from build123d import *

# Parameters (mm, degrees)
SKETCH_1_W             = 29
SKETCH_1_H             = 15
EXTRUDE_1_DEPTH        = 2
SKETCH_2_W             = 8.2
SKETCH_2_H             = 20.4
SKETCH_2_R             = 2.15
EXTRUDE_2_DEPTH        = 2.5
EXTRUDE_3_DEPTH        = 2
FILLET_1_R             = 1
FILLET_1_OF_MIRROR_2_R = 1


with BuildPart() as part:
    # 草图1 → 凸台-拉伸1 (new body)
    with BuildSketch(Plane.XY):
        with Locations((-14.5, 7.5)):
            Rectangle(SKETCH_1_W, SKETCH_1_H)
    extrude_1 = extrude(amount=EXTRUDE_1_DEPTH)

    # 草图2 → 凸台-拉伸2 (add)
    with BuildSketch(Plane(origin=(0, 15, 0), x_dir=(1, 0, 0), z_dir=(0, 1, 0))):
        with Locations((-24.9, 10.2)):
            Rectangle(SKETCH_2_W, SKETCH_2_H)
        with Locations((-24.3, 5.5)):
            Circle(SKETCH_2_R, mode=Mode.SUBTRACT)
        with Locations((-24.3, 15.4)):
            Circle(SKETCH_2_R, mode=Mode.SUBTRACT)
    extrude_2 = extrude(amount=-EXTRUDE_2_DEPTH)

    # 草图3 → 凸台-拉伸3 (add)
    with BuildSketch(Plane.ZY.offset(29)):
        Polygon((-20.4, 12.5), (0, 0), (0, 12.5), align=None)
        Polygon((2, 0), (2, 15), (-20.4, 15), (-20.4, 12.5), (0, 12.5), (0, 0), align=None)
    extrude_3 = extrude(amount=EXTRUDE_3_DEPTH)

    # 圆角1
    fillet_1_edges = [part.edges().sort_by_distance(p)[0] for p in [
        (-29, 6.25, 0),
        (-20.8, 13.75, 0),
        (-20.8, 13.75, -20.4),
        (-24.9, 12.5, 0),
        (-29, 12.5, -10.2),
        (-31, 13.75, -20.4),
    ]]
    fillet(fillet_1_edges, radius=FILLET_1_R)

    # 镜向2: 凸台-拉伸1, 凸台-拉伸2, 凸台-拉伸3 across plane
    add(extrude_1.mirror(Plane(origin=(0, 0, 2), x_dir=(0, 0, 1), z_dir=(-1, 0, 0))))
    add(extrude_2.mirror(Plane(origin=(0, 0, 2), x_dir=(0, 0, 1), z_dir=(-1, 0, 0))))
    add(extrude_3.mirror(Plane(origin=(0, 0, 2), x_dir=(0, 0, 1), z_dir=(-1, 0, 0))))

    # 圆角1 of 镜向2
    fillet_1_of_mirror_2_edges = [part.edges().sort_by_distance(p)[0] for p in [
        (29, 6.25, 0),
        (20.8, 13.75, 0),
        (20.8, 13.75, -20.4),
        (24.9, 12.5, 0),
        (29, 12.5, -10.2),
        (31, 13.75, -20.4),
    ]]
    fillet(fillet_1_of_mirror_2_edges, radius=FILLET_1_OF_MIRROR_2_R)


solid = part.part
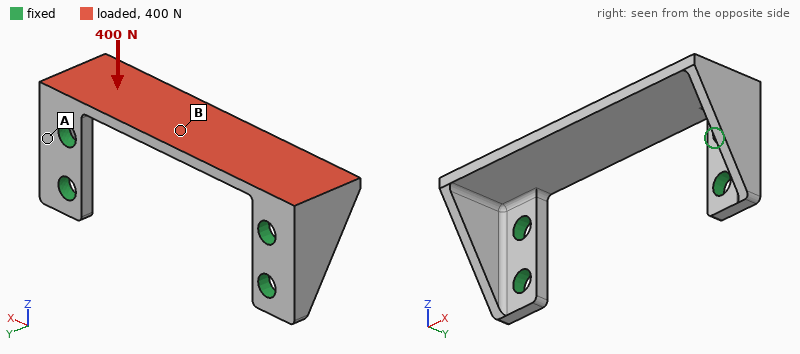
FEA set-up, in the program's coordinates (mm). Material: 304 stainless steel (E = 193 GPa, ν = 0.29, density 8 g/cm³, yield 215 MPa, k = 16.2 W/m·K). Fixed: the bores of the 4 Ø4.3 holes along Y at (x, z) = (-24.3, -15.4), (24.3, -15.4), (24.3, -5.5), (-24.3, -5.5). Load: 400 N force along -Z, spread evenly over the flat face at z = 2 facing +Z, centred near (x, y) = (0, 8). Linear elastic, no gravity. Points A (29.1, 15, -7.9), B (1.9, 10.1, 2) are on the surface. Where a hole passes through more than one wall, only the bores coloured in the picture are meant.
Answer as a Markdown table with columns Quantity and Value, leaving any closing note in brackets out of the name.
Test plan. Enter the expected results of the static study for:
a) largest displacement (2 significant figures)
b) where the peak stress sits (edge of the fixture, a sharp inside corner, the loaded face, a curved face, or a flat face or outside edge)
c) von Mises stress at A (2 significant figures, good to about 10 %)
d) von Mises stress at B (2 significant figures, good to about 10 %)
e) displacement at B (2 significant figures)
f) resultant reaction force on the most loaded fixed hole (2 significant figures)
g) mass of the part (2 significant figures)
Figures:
| Quantity | Value |
|---|---|
| largest displacement | 83 µm |
| where the peak stress sits | a curved face |
| von Mises stress at A | 18 MPa |
| von Mises stress at B | 68 MPa |
| displacement at B | 54 µm |
| resultant reaction force on the most loaded fixed hole | 220 N |
| mass of the part | 26 g |
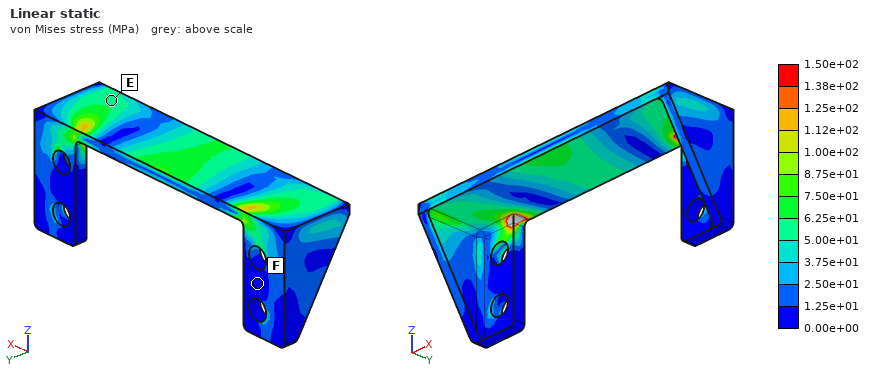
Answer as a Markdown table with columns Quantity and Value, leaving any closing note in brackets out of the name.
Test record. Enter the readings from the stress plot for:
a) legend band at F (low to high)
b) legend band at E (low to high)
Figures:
| Quantity | Value |
|---|---|
| legend band at F | 0.00e+00 to 1.25e+01 MPa |
| legend band at E | 5.00e+01 to 6.25e+01 MPa |
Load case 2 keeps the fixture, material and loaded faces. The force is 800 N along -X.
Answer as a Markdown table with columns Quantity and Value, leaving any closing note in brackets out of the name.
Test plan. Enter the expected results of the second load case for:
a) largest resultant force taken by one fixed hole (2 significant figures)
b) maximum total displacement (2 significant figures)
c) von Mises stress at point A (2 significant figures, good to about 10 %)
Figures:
| Quantity | Value |
|---|---|
| largest resultant force taken by one fixed hole | 490 N |
| maximum total displacement | 6.3 µm |
| von Mises stress at point A | 24 MPa |
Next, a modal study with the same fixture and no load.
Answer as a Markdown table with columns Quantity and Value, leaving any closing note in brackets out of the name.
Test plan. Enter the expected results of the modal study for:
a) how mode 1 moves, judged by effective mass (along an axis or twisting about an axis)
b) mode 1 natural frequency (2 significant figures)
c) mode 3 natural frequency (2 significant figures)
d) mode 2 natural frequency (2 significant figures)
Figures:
| Quantity | Value |
|---|---|
| how mode 1 moves, judged by effective mass | along Z |
| mode 1 natural frequency | 3700 Hz |
| mode 3 natural frequency | 8900 Hz |
| mode 2 natural frequency | 8500 Hz |
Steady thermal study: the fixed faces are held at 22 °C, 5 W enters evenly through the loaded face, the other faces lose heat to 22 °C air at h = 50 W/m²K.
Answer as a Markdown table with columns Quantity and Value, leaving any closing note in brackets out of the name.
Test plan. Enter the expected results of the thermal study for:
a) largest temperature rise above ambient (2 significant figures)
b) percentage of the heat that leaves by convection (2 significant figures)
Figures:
| Quantity | Value |
|---|---|
| largest temperature rise above ambient | 45 K |
| percentage of the heat that leaves by convection | 44 % |
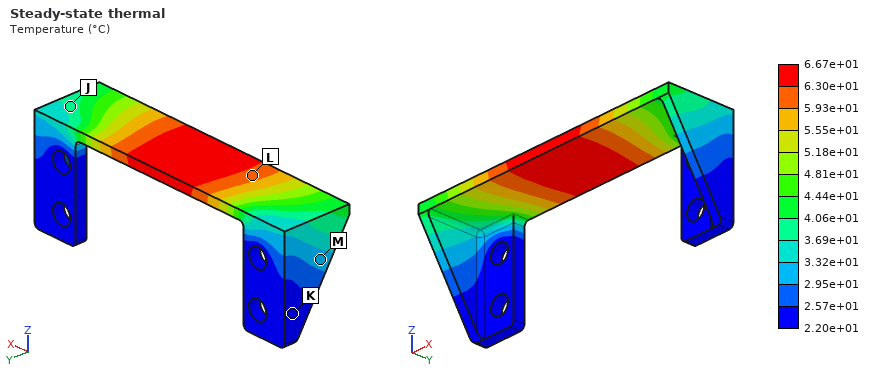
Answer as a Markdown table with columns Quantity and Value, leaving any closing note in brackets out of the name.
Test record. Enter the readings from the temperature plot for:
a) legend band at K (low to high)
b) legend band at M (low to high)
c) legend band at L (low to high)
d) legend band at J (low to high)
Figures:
| Quantity | Value |
|---|---|
| legend band at K | 2.20e+01 to 2.57e+01 °C |
| legend band at M | 2.95e+01 to 3.32e+01 °C |
| legend band at L | 5.93e+01 to 6.30e+01 °C |
| legend band at J | 3.69e+01 to 4.06e+01 °C |
